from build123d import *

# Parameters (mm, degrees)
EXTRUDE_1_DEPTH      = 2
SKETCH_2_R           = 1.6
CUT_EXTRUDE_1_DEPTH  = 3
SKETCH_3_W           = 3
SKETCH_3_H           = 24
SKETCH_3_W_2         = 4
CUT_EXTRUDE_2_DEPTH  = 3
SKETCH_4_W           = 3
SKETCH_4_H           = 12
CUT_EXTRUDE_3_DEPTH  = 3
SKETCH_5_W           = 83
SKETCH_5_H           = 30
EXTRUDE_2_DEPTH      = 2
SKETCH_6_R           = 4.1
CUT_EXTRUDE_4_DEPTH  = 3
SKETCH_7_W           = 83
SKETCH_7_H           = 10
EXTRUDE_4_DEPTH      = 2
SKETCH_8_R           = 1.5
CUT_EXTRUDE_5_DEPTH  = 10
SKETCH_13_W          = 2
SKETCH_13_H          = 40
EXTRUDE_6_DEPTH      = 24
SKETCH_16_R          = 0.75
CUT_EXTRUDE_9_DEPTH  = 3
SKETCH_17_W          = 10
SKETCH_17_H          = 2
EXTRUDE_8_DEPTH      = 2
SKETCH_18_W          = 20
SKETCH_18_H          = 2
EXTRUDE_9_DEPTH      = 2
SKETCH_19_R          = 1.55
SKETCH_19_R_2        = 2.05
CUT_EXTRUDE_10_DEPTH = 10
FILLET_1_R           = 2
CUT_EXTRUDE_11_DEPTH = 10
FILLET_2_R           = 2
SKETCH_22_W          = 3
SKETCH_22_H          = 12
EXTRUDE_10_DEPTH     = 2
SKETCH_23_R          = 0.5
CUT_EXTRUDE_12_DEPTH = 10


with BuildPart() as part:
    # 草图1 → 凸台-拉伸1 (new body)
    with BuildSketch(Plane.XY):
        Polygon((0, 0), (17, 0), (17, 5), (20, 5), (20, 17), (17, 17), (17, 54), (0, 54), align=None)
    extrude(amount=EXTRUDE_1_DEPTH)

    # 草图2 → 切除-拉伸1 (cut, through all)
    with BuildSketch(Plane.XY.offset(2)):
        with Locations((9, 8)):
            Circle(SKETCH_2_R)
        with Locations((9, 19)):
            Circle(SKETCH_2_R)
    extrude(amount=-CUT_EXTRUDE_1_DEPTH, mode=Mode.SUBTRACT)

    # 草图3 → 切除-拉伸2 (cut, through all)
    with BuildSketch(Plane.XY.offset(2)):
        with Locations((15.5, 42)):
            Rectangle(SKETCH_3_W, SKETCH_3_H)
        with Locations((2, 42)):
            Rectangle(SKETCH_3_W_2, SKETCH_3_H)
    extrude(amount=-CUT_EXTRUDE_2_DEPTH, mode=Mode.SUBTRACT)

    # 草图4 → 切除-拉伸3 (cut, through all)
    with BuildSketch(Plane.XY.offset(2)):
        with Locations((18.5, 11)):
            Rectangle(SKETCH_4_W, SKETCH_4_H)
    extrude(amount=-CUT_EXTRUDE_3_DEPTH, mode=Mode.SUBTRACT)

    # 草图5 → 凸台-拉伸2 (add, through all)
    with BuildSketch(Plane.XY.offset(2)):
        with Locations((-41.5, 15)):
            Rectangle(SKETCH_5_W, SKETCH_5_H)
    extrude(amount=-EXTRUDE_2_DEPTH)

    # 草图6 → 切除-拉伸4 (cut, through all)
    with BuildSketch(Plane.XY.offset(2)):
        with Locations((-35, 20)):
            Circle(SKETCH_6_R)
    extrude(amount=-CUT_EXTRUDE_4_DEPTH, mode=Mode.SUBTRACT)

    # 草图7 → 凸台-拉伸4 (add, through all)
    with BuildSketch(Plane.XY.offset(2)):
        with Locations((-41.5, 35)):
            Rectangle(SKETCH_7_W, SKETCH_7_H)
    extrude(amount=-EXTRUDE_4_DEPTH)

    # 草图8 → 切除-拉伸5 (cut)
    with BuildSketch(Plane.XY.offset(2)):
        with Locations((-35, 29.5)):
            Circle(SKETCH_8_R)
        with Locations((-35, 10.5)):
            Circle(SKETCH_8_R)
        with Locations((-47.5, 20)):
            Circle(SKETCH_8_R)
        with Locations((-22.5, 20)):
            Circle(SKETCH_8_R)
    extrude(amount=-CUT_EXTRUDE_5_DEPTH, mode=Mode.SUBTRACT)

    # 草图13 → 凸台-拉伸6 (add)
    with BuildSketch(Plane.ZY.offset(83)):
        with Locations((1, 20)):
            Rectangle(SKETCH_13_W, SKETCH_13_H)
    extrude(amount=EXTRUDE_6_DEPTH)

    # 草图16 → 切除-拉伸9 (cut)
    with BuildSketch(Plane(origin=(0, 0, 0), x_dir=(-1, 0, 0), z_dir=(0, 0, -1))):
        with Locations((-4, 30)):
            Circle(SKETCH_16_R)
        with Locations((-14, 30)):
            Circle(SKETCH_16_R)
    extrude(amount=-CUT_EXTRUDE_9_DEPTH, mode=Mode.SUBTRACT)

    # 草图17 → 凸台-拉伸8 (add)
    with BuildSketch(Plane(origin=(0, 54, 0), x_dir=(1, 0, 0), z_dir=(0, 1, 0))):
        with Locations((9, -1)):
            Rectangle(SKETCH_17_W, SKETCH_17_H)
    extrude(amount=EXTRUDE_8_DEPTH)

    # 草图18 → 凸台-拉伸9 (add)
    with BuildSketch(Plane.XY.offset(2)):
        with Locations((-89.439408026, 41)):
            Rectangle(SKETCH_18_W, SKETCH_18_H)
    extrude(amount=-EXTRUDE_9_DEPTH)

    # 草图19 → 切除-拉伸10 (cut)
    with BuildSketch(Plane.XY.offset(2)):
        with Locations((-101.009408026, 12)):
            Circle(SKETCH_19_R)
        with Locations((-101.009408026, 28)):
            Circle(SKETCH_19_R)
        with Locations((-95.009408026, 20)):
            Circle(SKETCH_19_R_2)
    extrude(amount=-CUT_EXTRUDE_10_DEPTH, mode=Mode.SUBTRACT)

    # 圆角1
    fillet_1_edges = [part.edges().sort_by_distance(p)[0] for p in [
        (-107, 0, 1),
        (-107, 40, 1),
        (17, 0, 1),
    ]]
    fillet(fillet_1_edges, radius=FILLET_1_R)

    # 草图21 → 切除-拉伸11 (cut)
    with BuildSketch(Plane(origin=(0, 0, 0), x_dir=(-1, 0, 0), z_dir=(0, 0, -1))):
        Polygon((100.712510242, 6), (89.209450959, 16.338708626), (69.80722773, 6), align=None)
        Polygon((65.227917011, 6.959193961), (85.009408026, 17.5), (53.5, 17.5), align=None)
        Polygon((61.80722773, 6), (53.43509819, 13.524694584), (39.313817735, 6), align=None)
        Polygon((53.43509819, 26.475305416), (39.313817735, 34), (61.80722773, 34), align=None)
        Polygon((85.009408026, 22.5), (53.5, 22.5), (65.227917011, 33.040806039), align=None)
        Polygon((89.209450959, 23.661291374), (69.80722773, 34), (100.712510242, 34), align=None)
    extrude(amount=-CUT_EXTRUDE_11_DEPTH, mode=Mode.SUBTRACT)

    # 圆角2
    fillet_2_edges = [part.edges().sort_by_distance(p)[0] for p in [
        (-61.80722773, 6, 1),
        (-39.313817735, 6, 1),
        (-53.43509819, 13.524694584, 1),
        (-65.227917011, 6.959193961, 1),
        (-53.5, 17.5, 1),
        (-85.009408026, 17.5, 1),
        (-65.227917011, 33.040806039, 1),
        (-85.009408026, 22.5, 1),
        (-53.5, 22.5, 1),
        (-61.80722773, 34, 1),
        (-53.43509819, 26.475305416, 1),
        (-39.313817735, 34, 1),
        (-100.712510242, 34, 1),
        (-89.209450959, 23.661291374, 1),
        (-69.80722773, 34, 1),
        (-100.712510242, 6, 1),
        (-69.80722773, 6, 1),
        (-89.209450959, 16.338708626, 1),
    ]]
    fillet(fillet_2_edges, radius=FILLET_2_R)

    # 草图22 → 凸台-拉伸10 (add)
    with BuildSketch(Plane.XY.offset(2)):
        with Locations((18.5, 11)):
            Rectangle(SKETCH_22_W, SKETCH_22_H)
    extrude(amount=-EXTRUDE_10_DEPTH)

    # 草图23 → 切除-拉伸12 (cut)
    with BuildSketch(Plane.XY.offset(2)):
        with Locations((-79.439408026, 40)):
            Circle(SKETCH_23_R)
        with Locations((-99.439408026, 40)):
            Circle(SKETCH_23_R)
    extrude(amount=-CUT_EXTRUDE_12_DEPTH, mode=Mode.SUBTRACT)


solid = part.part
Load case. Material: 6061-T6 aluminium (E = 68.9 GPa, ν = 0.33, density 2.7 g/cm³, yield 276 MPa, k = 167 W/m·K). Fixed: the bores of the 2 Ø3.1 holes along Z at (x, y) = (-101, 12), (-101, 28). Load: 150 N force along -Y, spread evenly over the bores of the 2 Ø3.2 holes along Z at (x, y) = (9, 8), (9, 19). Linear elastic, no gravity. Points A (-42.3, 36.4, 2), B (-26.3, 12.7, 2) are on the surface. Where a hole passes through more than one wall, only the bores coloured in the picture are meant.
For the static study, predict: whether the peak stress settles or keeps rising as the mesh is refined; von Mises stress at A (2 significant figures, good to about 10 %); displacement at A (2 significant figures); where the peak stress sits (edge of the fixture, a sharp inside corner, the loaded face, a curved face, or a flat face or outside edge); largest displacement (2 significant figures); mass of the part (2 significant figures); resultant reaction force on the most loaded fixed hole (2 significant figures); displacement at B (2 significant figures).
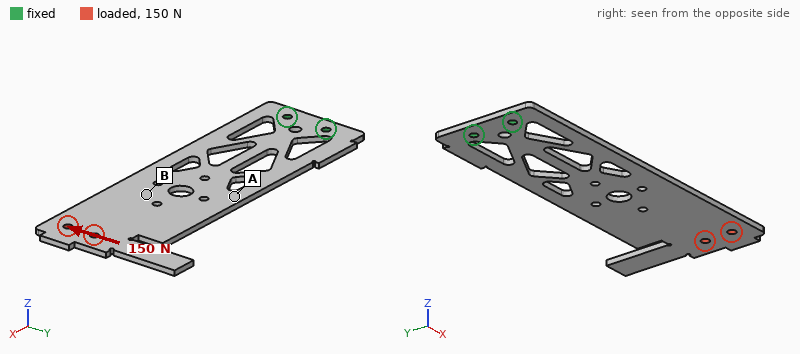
keeps rising
17 MPa
0.13 mm
edge of the fixture
0.30 mm
23 g
840 N
0.17 mm
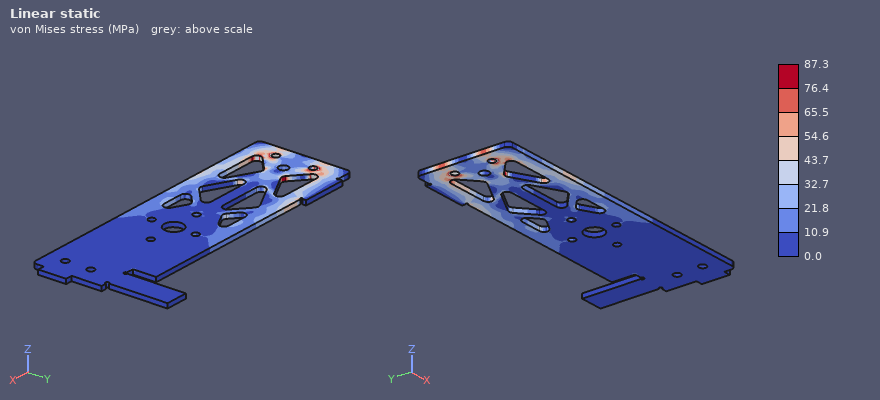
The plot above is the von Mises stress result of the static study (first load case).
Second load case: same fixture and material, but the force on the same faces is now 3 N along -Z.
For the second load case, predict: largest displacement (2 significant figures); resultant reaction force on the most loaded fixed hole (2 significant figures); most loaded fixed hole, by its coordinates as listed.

1.4 mm
2.2 N
(-101, 12)
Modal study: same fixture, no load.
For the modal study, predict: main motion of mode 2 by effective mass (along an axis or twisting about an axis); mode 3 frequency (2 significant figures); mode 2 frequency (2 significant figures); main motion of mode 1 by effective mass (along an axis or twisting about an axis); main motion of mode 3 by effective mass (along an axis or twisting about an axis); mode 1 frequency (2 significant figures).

twisting about X
660 Hz
460 Hz
along Z
along Z
89 Hz
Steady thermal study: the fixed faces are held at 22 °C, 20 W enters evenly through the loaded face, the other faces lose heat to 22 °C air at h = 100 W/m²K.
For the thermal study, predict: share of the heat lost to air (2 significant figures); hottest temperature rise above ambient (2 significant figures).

94 %
59 K
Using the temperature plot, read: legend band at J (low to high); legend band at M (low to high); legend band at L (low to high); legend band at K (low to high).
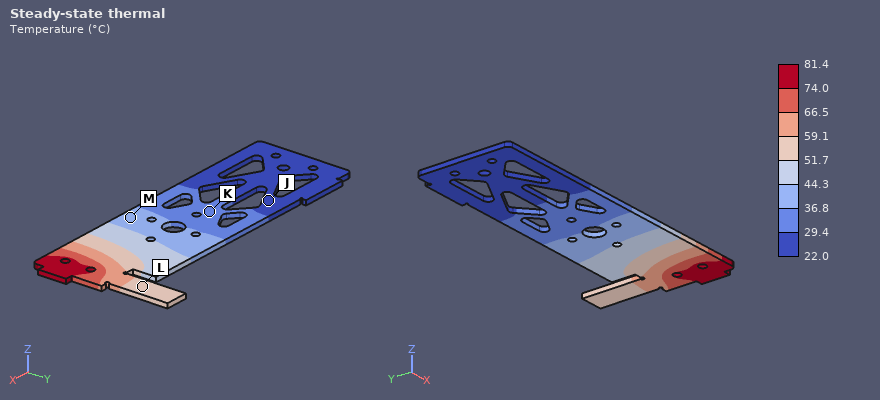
22.0 to 29.4 °C
36.8 to 44.3 °C
51.7 to 59.1 °C
29.4 to 36.8 °C
